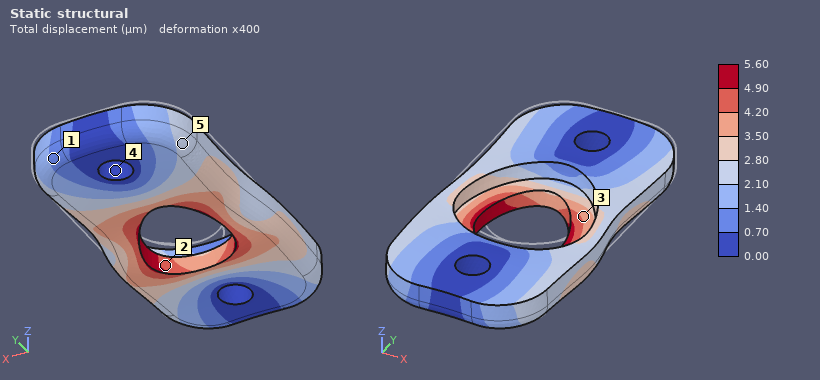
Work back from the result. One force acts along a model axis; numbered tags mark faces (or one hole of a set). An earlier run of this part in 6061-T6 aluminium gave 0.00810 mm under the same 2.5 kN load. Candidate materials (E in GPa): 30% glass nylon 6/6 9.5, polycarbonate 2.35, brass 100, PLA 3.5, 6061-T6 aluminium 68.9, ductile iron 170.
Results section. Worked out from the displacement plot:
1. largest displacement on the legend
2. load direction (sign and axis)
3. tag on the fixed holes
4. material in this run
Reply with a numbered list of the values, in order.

1. 5.60 µm
2. -Y
3. 4
4. brass
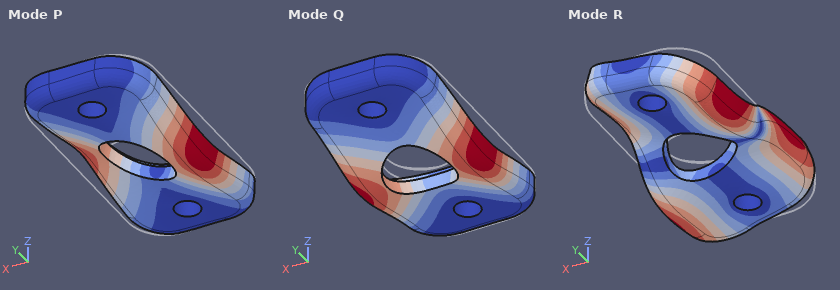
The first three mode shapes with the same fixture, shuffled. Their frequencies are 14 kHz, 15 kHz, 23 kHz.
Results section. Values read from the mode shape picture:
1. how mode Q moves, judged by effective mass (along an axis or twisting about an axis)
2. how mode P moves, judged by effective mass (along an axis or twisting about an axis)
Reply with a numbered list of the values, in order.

1. along Z
2. twisting about Y
